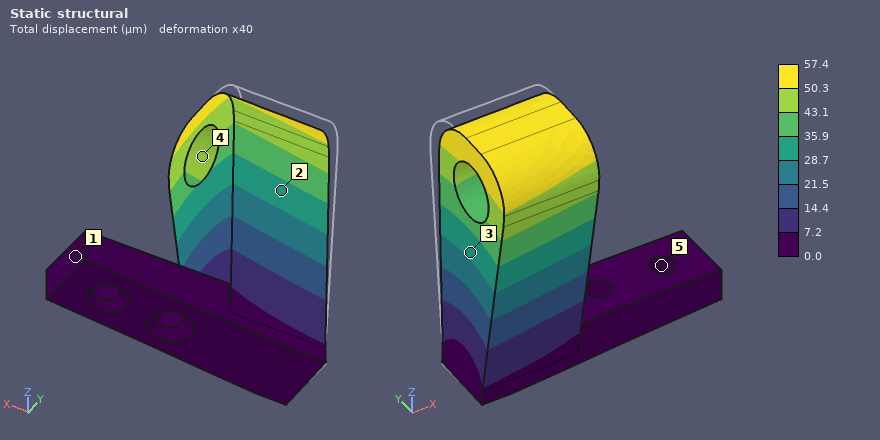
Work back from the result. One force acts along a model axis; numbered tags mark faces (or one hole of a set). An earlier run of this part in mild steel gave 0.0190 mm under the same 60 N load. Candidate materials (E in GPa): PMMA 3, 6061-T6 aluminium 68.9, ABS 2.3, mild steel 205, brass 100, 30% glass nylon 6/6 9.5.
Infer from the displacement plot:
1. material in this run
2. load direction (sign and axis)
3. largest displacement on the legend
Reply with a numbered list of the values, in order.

1. 6061-T6 aluminium
2. -Y
3. 57.4 µm
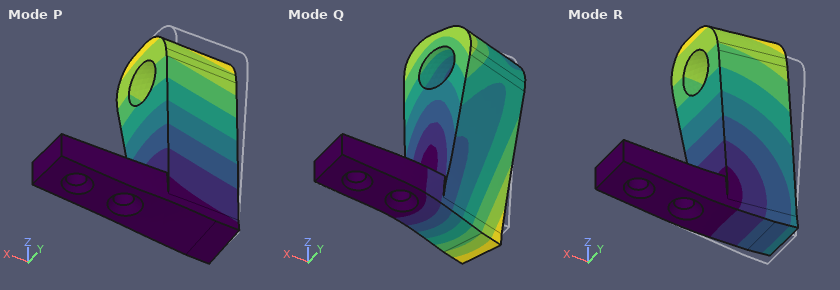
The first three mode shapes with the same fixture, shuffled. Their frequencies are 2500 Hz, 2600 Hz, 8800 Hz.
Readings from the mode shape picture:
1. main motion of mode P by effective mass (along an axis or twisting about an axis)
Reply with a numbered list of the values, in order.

1. along Y
